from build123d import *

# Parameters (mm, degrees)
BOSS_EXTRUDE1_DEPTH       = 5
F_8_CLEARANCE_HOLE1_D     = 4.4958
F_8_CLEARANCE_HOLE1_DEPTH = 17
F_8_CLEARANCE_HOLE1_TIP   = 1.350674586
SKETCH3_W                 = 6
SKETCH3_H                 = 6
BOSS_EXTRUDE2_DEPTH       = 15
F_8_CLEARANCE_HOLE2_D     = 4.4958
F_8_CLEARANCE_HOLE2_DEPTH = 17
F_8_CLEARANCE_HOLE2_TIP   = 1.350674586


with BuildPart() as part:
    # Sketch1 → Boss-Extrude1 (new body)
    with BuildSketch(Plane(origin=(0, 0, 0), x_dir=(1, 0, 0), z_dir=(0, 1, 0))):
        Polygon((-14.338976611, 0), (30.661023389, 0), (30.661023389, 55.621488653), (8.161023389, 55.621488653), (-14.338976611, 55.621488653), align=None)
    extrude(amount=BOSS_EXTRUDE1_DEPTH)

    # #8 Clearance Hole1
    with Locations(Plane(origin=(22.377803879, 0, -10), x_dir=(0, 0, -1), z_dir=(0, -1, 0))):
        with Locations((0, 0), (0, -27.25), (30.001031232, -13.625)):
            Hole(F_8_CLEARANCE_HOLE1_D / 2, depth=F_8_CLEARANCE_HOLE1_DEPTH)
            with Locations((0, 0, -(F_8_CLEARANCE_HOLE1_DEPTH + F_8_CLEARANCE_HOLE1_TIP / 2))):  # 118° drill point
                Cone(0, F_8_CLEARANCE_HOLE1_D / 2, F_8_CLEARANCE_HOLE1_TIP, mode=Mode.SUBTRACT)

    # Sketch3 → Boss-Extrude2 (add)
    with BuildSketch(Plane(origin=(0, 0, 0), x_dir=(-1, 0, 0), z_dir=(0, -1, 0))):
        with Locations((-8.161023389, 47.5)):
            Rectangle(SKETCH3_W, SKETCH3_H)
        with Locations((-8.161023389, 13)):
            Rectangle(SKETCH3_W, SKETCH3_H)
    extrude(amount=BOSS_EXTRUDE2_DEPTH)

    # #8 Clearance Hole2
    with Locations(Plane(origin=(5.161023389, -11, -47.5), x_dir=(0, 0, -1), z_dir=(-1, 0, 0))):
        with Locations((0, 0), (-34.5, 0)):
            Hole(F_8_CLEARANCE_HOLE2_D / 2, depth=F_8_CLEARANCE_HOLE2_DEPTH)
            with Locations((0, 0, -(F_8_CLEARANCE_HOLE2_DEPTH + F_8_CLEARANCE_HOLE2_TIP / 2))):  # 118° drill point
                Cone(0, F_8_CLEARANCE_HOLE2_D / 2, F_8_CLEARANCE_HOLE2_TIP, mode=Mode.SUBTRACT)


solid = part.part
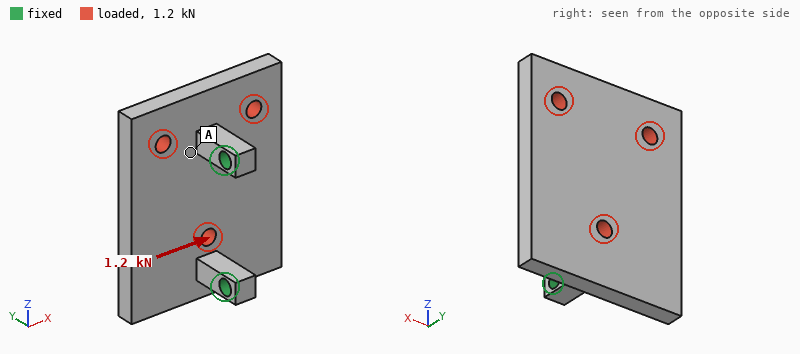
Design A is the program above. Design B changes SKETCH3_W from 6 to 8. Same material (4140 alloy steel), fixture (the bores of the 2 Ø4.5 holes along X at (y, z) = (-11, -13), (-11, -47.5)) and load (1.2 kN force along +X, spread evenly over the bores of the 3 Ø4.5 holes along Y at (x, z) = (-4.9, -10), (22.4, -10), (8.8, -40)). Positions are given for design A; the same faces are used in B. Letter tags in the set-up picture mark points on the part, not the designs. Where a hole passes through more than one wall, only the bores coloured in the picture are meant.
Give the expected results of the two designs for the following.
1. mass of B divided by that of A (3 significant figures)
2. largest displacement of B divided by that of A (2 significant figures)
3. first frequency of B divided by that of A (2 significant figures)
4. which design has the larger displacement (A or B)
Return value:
1.02
0.48
1.5
A
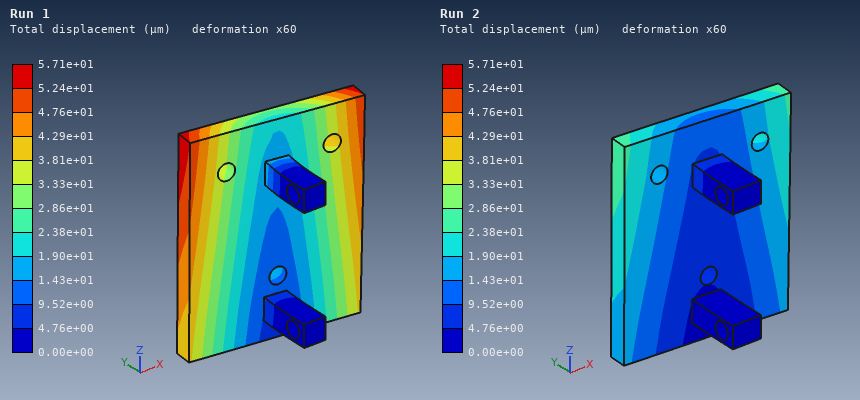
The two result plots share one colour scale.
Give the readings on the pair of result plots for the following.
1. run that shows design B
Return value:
Run 2
